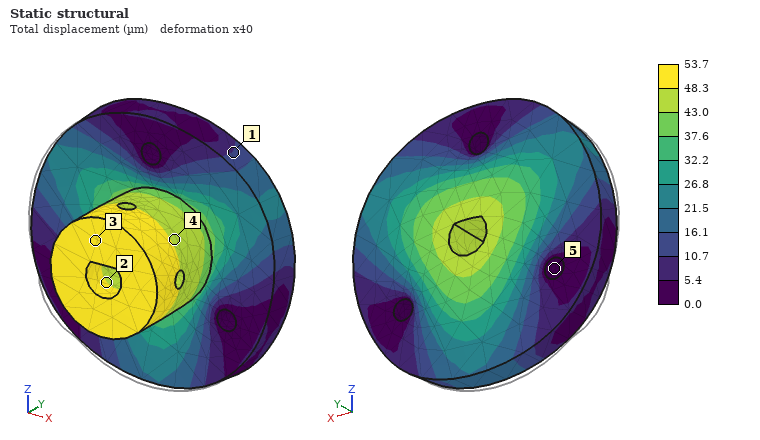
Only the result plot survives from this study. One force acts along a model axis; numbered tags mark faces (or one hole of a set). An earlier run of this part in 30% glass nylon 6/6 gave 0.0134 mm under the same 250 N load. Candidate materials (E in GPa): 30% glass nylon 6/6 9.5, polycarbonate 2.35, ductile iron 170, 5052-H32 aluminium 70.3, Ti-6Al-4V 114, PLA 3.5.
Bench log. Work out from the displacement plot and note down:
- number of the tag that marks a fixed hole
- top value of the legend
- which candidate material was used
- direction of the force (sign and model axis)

5
53.7 µm
polycarbonate
+Y
